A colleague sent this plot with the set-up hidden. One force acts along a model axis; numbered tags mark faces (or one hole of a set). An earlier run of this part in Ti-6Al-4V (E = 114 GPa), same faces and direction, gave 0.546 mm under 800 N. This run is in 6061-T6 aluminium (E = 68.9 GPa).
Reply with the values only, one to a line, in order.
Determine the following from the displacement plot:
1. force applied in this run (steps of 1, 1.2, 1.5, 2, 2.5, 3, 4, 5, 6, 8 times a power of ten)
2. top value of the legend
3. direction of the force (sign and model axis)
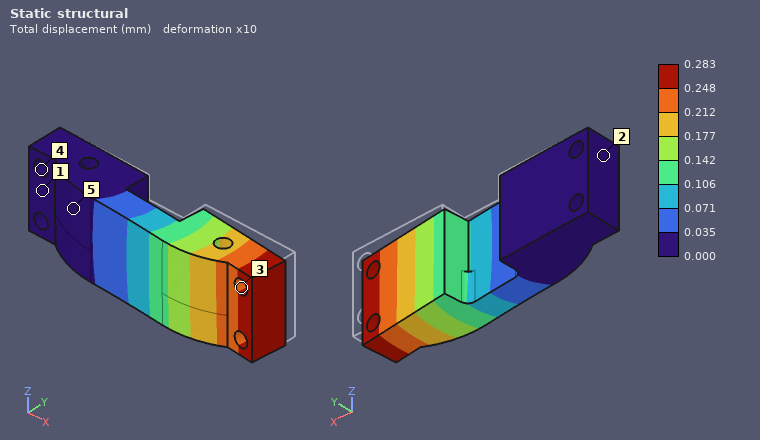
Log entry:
250 N
0.283 mm
-Y
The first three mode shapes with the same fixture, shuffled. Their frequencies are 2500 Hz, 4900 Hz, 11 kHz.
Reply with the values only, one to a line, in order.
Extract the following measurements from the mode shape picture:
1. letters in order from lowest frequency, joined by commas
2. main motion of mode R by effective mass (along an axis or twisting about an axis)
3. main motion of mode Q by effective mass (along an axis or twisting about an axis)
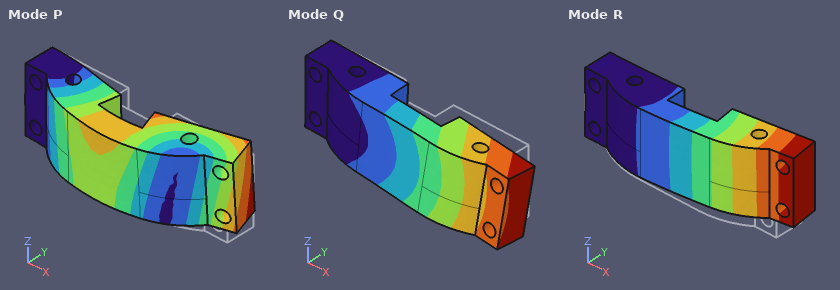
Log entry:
R, Q, P
along Y
along Z
